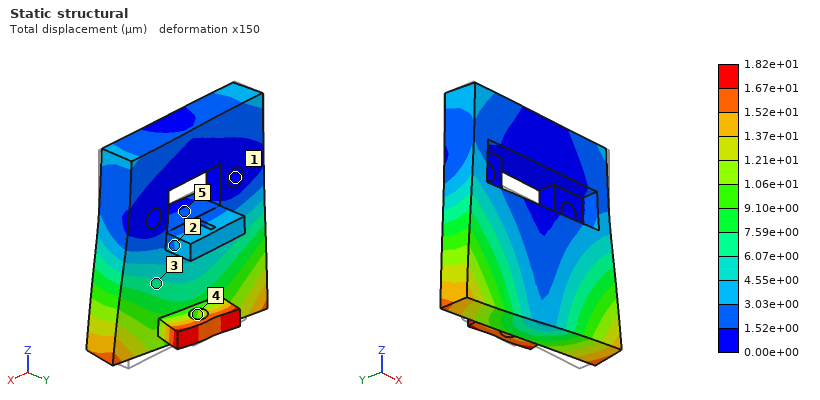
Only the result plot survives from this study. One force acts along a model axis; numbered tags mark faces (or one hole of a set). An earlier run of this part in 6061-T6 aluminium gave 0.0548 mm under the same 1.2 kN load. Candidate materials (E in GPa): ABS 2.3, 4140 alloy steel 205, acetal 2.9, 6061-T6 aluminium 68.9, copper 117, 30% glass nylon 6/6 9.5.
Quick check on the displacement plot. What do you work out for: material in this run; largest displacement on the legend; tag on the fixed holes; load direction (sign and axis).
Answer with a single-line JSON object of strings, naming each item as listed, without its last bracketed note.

{"material in this run": "4140 alloy steel", "largest displacement on the legend": "1.82e+01 µm", "tag on the fixed holes": "1", "load direction": "+X"}
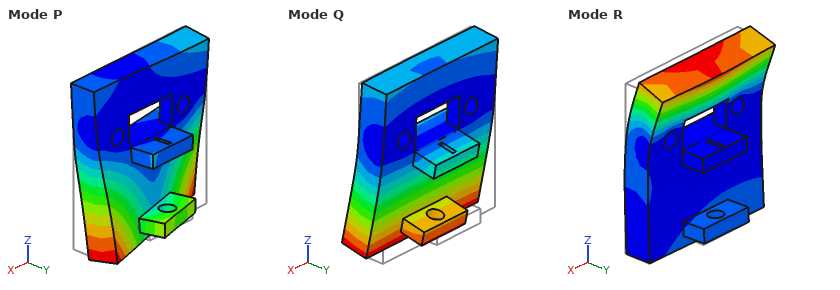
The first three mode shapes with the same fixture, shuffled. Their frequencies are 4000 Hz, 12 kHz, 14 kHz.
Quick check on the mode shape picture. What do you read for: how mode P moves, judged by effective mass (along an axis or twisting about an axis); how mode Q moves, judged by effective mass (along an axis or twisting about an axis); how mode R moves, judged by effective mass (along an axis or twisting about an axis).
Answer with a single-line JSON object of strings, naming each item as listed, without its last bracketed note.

{"how mode P moves, judged by effective mass": "twisting about Z", "how mode Q moves, judged by effective mass": "along Y", "how mode R moves, judged by effective mass": "along Y"}
